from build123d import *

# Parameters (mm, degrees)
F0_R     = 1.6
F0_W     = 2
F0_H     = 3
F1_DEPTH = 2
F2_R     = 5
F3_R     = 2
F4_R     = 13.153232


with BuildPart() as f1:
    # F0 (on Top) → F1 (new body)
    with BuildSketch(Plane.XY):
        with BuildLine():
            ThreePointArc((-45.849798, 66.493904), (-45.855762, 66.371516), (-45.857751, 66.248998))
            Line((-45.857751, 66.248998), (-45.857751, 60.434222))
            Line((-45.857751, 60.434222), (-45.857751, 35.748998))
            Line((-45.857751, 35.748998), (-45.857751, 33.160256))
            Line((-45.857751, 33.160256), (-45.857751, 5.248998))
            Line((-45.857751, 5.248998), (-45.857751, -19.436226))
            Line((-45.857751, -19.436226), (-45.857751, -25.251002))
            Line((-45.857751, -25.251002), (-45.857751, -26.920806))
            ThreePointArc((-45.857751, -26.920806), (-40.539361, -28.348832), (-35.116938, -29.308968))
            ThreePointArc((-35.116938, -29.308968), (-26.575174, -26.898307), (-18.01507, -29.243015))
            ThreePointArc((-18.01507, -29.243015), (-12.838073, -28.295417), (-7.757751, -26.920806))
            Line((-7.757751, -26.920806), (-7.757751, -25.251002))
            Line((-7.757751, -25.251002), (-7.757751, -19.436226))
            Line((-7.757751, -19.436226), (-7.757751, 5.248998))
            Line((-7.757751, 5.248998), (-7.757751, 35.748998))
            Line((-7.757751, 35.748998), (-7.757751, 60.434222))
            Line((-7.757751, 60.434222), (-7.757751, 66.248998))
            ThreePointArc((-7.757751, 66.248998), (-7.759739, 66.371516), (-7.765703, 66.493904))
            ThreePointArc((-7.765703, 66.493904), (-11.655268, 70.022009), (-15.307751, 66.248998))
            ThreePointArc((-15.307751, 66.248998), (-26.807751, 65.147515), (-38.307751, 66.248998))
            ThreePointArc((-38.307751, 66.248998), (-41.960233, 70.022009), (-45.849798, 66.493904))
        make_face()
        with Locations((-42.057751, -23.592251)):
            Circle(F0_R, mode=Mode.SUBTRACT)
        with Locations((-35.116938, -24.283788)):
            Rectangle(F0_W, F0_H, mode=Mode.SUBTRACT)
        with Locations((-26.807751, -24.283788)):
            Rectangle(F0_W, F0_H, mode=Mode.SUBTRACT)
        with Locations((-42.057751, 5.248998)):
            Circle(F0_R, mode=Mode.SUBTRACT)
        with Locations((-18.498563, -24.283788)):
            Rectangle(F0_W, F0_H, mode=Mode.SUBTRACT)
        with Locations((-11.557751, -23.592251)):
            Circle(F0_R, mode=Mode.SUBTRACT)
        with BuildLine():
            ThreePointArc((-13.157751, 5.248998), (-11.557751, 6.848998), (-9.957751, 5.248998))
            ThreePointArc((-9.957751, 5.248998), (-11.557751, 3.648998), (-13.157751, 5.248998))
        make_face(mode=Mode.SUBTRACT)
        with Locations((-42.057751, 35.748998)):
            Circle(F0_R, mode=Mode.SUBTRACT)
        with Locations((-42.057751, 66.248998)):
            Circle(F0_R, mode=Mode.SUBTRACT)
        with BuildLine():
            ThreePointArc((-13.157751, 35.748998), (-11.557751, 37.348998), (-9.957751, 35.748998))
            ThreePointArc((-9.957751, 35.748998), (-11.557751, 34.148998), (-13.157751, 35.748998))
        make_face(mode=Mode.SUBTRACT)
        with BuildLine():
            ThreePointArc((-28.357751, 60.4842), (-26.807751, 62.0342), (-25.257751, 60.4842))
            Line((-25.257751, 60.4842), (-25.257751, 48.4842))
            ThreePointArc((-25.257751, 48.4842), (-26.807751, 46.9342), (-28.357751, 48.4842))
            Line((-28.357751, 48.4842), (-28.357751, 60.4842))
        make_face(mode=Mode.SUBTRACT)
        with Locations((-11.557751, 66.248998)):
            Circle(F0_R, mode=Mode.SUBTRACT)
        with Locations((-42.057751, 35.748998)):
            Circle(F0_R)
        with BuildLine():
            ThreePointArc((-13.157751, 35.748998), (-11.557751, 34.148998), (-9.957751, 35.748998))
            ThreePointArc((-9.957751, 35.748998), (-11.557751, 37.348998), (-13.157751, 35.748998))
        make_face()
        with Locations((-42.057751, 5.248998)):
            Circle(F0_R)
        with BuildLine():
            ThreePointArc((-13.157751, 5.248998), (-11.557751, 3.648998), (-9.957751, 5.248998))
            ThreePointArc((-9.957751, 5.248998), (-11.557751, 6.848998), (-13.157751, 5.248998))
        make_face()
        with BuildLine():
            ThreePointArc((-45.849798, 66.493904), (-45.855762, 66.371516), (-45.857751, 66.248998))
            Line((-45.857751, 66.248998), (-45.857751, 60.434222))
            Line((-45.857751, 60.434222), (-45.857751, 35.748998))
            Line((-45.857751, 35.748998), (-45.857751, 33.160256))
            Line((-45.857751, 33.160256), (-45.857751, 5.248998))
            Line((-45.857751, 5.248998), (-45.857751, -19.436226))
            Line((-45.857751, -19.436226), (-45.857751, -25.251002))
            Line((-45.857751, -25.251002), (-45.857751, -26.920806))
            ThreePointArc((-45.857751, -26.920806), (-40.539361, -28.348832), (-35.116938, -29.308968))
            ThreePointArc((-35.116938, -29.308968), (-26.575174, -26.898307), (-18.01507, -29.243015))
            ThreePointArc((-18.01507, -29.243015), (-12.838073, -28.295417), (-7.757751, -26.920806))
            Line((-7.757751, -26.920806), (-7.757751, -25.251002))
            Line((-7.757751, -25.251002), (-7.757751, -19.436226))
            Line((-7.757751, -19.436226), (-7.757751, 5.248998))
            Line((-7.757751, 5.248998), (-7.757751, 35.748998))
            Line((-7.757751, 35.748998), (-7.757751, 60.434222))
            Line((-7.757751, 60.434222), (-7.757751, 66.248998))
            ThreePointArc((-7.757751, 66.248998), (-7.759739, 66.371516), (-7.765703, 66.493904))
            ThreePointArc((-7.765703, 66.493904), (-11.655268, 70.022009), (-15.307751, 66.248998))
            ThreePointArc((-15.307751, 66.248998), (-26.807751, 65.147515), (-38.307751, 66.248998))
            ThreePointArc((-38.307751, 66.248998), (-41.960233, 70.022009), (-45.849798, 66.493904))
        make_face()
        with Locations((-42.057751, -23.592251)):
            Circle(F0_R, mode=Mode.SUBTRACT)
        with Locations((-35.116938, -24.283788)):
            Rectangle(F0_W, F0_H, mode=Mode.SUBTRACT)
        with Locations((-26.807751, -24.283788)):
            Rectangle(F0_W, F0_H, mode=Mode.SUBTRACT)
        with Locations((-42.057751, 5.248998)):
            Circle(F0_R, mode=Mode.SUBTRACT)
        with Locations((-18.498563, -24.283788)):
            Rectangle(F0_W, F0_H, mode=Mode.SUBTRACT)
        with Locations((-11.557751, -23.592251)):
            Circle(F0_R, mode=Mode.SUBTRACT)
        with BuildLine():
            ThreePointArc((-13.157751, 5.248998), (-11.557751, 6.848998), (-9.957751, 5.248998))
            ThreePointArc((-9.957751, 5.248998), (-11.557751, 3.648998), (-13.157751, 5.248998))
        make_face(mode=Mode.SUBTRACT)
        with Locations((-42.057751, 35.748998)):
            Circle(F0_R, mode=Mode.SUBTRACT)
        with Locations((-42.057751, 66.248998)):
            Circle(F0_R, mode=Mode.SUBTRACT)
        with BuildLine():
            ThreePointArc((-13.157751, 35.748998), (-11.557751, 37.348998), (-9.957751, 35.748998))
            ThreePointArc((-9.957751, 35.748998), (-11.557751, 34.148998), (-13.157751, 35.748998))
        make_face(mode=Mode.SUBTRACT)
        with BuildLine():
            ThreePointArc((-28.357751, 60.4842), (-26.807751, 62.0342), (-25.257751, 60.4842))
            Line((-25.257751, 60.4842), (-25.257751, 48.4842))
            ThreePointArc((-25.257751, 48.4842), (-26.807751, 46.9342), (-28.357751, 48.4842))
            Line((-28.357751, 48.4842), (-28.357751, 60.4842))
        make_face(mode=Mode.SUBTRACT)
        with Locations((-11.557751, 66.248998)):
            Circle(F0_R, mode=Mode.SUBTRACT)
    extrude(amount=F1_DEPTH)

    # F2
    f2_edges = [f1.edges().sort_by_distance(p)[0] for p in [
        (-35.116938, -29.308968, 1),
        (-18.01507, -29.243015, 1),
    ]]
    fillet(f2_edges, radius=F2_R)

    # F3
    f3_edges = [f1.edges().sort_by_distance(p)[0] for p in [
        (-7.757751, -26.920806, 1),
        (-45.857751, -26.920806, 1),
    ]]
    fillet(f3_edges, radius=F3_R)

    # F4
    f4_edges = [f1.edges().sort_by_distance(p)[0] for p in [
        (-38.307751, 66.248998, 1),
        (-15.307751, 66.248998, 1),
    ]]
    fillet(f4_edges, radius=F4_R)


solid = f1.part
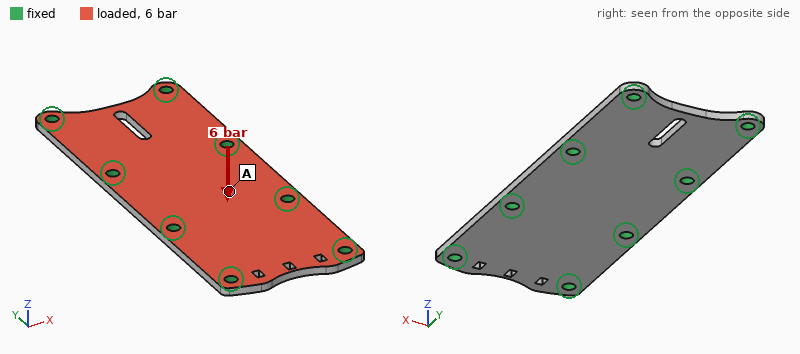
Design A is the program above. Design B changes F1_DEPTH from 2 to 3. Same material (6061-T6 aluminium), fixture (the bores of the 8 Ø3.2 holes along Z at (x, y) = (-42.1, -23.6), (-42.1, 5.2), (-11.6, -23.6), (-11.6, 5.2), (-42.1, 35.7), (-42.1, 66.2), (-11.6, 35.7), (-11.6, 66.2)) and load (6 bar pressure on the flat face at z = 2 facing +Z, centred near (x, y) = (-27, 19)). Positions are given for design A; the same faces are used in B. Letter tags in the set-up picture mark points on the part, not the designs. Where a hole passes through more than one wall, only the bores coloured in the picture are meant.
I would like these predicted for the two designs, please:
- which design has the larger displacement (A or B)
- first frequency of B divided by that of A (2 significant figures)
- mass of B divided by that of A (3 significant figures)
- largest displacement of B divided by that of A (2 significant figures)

A
1.4
1.50
0.33
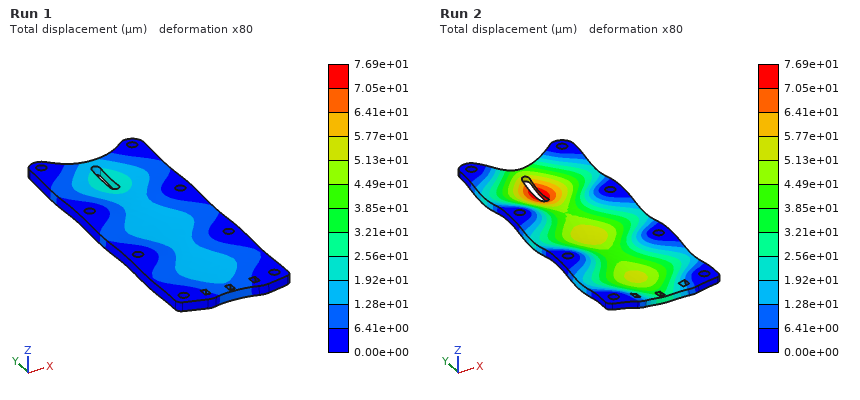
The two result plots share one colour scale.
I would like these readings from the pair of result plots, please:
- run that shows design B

Run 1
